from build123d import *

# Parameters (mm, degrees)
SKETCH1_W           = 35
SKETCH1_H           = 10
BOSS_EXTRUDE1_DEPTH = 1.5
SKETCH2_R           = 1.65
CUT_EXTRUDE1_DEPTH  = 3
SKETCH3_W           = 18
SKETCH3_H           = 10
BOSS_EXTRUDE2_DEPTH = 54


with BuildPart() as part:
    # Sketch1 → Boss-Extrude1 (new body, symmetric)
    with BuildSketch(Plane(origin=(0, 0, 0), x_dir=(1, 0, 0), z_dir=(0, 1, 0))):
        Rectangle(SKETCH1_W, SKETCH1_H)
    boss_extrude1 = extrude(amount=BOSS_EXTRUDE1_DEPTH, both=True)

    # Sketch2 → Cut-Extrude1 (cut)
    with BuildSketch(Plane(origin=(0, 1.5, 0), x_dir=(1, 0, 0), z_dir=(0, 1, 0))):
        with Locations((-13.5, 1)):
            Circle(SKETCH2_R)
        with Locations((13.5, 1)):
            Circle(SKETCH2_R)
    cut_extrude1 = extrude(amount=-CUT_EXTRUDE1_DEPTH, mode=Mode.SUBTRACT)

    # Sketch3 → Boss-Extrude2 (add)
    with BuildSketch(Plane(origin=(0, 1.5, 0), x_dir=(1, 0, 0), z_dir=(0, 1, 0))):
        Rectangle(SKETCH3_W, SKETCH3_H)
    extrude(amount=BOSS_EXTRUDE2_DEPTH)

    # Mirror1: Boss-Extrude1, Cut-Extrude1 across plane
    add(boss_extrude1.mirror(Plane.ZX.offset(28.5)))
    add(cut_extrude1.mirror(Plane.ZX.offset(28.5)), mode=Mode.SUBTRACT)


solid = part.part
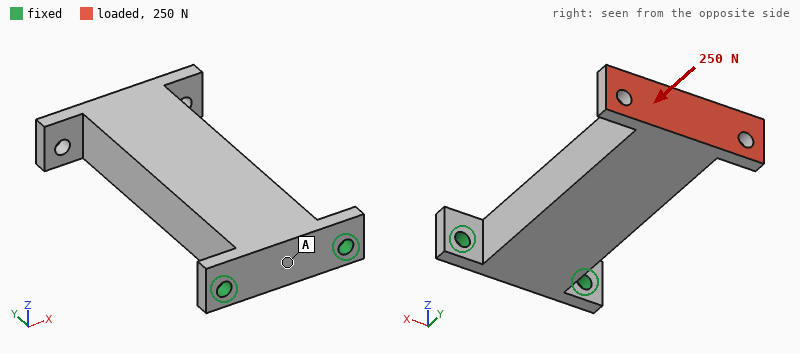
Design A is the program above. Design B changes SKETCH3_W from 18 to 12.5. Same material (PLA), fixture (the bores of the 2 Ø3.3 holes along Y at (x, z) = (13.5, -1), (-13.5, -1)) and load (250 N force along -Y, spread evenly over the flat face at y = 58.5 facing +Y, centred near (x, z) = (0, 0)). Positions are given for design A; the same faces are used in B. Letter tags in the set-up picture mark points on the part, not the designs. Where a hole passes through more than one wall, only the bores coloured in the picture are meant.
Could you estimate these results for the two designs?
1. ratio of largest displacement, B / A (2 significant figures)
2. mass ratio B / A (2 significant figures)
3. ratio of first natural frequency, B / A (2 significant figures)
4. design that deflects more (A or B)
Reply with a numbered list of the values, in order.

1. 1.8
2. 0.75
3. 0.90
4. B
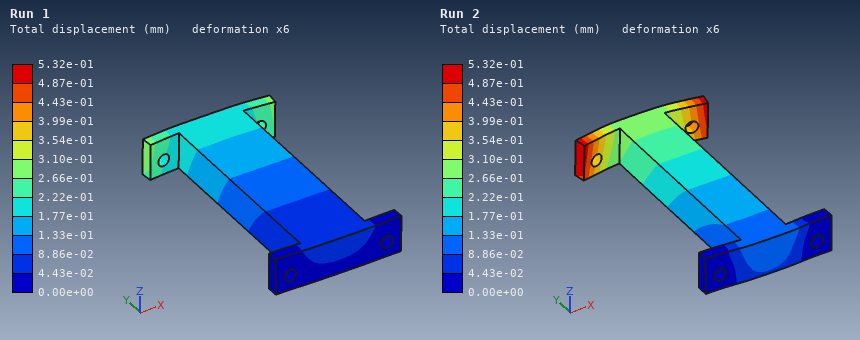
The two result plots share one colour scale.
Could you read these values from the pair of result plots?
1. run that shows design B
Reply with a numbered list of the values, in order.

1. Run 2
